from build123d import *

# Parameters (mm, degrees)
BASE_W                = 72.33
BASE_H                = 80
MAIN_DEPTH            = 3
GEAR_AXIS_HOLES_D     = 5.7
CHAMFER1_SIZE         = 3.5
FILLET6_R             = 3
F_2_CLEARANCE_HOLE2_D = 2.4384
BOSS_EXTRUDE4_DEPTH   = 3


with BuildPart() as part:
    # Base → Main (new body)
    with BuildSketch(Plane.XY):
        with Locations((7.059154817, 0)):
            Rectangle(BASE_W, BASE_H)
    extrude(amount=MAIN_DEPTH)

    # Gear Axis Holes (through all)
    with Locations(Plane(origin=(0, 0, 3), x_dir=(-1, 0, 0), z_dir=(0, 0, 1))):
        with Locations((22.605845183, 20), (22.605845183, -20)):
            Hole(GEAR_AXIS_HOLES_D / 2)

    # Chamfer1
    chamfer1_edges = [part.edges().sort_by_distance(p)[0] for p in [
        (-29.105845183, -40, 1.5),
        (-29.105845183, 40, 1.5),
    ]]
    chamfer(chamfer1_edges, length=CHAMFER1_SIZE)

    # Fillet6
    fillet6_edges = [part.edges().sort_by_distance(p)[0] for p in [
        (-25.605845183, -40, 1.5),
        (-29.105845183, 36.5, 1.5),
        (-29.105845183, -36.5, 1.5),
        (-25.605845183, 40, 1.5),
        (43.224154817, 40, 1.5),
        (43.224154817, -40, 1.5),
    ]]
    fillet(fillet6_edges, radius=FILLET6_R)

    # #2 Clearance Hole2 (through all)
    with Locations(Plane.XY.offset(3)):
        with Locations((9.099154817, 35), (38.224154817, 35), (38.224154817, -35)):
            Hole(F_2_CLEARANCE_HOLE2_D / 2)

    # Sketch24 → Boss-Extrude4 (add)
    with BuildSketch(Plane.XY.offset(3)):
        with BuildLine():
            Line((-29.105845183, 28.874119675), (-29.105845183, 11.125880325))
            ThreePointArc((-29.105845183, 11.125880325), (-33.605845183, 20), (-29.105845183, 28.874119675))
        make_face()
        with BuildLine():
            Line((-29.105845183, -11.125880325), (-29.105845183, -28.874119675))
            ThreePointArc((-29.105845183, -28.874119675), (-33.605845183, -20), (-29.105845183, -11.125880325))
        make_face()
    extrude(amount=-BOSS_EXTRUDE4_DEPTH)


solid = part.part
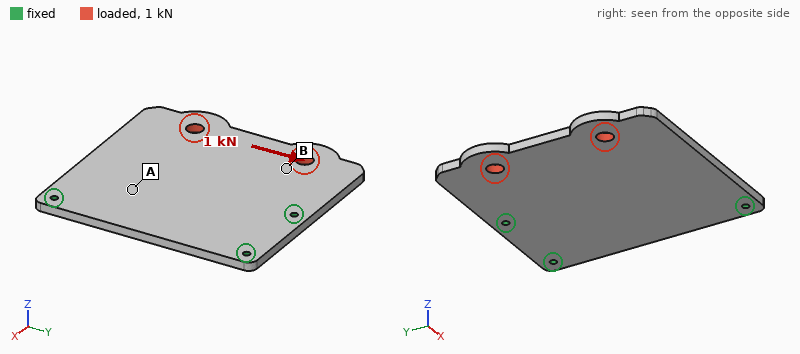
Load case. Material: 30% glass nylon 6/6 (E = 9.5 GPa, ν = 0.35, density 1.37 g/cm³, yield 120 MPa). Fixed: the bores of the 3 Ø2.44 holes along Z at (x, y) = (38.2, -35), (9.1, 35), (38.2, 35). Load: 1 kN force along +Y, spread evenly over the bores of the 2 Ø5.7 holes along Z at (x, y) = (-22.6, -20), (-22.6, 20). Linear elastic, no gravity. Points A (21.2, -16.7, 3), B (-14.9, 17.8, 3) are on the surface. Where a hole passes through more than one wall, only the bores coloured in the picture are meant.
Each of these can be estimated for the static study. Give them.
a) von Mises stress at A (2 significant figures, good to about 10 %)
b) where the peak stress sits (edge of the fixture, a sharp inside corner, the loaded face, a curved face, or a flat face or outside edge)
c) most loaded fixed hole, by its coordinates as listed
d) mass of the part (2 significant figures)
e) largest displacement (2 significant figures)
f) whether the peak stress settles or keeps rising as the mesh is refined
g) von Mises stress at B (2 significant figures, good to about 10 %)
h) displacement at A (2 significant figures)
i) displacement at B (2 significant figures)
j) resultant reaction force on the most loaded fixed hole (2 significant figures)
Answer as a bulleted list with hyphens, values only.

- 5.0 MPa
- edge of the fixture
- (9.1, 35)
- 24 g
- 0.12 mm
- keeps rising
- 11 MPa
- 0.025 mm
- 0.077 mm
- 820 N
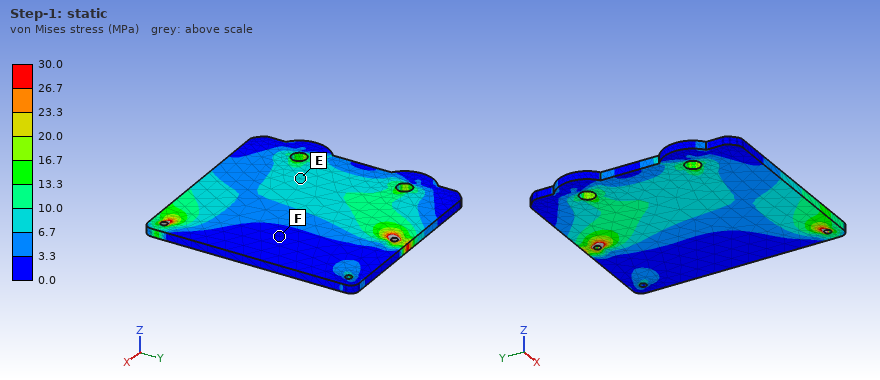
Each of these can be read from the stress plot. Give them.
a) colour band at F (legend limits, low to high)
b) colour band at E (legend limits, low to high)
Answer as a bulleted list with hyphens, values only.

- 0.0 to 3.3 MPa
- 6.7 to 10.0 MPa
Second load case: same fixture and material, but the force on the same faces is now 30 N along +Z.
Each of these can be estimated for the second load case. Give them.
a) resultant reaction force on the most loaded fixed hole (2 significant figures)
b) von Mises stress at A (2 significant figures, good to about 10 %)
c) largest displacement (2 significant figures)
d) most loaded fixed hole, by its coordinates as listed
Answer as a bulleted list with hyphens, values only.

- 39 N
- 5.2 MPa
- 1.2 mm
- (9.1, 35)
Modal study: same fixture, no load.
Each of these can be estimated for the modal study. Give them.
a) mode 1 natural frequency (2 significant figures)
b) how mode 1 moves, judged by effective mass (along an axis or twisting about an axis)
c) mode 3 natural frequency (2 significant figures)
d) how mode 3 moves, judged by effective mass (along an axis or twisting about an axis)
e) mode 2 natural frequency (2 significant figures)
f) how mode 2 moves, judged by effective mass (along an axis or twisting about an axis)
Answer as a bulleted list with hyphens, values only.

- 350 Hz
- along Z
- 1400 Hz
- along Z
- 920 Hz
- twisting about X
